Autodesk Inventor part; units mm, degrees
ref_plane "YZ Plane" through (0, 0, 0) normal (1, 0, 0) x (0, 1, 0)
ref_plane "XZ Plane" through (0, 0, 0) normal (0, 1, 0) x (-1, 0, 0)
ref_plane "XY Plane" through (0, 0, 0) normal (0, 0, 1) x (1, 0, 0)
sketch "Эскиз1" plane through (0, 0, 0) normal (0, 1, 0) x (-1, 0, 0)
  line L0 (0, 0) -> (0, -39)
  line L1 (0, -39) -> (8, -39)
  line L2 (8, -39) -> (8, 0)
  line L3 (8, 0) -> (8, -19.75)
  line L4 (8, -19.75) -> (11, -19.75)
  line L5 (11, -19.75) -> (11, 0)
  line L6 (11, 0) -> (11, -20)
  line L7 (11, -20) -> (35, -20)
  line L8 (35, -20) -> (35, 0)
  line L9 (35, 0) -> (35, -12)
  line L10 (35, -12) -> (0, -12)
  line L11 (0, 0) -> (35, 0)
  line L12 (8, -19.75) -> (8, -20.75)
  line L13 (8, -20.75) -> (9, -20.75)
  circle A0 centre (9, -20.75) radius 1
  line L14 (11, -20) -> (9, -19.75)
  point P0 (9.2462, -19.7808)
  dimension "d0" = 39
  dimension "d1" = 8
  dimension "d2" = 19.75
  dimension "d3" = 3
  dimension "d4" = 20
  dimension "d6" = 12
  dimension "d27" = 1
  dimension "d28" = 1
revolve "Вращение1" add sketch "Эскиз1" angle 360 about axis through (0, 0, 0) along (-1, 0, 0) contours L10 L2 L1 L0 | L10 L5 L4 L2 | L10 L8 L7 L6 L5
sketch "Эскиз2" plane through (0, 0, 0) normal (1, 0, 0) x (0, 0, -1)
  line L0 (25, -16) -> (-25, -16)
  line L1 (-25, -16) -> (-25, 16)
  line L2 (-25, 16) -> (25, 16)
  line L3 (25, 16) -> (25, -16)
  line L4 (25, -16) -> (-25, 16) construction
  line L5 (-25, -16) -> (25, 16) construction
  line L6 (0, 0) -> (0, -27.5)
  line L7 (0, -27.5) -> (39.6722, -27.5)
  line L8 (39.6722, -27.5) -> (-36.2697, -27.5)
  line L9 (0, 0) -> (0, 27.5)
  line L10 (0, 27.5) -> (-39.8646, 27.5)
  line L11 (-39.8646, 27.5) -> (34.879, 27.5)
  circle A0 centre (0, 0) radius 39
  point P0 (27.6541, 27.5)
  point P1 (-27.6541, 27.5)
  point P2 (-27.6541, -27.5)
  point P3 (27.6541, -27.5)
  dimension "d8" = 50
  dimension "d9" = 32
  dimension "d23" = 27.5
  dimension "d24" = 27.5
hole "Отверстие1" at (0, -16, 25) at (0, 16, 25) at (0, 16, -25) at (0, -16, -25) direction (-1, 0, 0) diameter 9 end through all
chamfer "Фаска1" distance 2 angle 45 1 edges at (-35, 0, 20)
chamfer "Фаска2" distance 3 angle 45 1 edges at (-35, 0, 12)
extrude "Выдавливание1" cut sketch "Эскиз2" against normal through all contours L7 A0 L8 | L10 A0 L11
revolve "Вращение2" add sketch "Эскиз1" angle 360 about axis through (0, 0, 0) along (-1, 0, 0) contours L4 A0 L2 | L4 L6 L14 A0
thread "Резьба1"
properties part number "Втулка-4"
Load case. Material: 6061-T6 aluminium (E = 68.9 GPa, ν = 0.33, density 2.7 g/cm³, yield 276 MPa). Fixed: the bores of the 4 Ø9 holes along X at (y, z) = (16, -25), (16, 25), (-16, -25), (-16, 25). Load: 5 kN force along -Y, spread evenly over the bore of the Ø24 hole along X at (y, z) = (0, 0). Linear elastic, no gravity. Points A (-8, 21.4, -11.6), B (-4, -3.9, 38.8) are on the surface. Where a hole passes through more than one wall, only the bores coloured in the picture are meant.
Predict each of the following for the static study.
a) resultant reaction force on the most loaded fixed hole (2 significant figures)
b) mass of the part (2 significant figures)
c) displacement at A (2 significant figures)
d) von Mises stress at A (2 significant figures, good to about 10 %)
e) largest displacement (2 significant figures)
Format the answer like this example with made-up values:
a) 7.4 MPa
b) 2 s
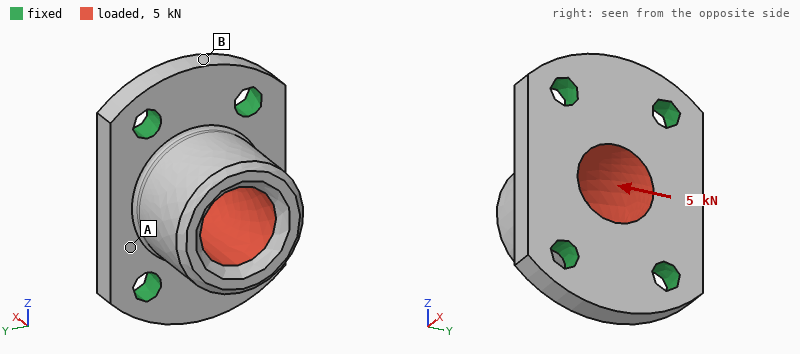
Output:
a) 1.7 kN
b) 130 g
c) 5.5 µm
d) 10 MPa
e) 18 µm
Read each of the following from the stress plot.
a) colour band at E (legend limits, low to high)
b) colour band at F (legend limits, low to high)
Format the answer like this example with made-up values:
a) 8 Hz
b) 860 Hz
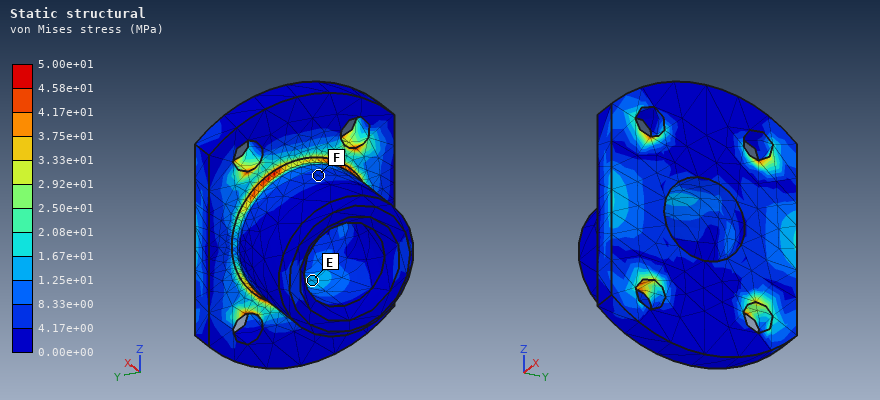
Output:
a) 1.25e+01 to 1.67e+01 MPa
b) 4.17e+00 to 8.33e+00 MPa
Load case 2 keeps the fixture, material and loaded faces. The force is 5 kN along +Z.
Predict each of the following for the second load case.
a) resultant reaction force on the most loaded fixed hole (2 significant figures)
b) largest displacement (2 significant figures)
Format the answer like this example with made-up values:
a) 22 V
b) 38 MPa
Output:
a) 1.5 kN
b) 11 µm
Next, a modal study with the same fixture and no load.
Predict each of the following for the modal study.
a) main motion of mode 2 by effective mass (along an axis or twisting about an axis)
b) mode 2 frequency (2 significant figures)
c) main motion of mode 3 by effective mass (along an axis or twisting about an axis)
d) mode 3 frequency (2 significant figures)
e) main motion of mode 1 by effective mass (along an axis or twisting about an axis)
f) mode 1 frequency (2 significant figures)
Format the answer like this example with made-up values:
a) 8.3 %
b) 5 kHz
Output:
a) along Z
b) 14 kHz
c) along X
d) 15 kHz
e) along Y
f) 10000 Hz
